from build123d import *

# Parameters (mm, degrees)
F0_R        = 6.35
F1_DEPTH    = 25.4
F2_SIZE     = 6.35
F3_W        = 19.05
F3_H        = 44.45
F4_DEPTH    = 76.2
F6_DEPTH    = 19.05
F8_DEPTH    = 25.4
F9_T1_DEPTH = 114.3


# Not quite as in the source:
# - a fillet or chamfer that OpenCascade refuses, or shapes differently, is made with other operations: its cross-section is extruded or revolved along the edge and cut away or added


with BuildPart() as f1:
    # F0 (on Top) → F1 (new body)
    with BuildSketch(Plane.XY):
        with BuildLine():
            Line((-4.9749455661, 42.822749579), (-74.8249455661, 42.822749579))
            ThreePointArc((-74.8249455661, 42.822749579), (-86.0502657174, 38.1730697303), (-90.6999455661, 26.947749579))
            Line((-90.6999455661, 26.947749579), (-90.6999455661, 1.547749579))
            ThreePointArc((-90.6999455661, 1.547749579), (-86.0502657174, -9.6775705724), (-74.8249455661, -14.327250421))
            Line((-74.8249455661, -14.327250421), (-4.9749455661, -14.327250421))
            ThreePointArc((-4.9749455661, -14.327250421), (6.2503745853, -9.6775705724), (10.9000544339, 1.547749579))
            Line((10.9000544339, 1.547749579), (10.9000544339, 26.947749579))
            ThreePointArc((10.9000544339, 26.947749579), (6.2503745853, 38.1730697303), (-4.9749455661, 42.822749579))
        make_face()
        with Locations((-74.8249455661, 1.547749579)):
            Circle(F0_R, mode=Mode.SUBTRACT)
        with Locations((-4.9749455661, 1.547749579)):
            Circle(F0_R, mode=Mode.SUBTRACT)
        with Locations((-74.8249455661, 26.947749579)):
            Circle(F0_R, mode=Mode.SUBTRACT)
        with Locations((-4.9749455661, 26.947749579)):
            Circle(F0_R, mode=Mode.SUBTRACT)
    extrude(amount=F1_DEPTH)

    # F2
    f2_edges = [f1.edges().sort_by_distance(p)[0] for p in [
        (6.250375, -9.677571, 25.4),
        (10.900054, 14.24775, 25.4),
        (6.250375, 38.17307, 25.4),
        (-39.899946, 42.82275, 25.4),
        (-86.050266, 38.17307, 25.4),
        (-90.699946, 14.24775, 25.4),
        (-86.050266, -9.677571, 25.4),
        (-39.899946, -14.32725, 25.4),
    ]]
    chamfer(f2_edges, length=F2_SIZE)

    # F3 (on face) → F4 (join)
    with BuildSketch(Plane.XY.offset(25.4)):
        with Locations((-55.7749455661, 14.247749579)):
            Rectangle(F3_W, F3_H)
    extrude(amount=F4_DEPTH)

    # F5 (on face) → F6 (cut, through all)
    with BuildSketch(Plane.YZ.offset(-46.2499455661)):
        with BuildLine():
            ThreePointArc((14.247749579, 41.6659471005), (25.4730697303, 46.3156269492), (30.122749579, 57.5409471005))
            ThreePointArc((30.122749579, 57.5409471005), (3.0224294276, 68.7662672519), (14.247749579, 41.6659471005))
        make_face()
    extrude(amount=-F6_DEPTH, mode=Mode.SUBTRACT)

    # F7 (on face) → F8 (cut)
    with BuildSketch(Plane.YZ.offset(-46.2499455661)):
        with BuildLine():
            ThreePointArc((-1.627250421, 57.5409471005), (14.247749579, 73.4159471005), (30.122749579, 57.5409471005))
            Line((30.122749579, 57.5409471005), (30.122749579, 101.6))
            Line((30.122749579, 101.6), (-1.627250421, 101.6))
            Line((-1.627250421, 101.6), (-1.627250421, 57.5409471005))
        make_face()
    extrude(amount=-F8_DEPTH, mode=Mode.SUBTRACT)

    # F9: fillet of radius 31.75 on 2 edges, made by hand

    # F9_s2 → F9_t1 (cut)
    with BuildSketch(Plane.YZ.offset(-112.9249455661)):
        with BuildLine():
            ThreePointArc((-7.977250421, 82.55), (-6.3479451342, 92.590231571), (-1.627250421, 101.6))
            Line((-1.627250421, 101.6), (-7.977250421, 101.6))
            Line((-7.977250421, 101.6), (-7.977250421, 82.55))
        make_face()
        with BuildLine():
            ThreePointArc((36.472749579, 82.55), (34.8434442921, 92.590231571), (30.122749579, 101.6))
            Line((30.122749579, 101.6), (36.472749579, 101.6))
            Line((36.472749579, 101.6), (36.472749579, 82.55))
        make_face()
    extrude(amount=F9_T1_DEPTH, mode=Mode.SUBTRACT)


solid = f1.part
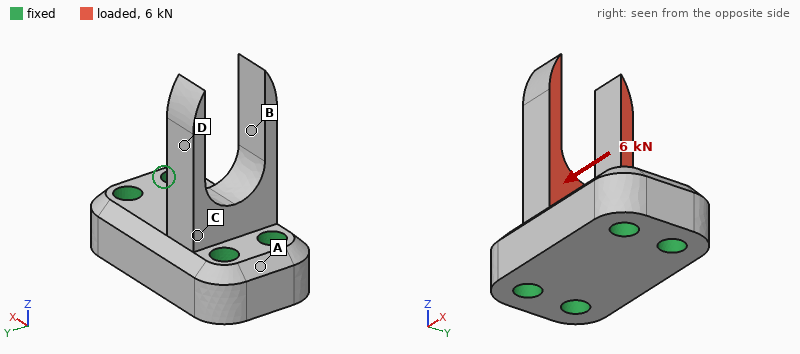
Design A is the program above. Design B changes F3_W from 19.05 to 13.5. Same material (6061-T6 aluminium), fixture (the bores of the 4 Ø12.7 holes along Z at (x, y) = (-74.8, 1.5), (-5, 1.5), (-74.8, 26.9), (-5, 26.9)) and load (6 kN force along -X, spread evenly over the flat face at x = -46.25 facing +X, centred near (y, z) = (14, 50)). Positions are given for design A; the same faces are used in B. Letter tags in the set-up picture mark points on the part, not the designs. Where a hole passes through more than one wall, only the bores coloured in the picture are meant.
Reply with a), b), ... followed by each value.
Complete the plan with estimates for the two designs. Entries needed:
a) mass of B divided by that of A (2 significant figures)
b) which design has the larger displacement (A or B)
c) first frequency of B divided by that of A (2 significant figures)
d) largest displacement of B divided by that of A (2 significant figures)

a) 0.94
b) B
c) 1.00
d) 2.4
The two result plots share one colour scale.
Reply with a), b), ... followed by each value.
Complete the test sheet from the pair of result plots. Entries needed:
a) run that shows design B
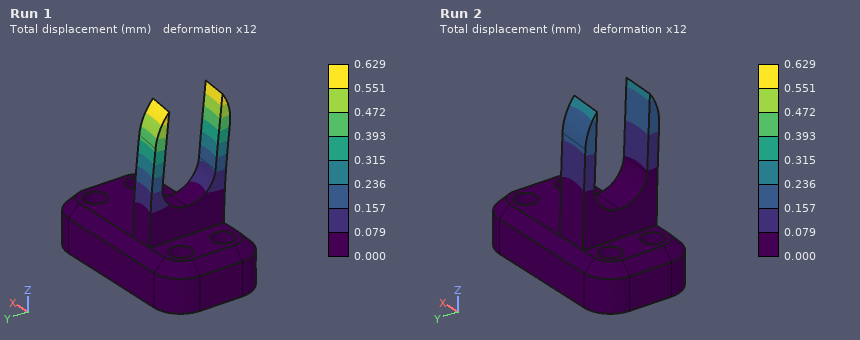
a) Run 1
